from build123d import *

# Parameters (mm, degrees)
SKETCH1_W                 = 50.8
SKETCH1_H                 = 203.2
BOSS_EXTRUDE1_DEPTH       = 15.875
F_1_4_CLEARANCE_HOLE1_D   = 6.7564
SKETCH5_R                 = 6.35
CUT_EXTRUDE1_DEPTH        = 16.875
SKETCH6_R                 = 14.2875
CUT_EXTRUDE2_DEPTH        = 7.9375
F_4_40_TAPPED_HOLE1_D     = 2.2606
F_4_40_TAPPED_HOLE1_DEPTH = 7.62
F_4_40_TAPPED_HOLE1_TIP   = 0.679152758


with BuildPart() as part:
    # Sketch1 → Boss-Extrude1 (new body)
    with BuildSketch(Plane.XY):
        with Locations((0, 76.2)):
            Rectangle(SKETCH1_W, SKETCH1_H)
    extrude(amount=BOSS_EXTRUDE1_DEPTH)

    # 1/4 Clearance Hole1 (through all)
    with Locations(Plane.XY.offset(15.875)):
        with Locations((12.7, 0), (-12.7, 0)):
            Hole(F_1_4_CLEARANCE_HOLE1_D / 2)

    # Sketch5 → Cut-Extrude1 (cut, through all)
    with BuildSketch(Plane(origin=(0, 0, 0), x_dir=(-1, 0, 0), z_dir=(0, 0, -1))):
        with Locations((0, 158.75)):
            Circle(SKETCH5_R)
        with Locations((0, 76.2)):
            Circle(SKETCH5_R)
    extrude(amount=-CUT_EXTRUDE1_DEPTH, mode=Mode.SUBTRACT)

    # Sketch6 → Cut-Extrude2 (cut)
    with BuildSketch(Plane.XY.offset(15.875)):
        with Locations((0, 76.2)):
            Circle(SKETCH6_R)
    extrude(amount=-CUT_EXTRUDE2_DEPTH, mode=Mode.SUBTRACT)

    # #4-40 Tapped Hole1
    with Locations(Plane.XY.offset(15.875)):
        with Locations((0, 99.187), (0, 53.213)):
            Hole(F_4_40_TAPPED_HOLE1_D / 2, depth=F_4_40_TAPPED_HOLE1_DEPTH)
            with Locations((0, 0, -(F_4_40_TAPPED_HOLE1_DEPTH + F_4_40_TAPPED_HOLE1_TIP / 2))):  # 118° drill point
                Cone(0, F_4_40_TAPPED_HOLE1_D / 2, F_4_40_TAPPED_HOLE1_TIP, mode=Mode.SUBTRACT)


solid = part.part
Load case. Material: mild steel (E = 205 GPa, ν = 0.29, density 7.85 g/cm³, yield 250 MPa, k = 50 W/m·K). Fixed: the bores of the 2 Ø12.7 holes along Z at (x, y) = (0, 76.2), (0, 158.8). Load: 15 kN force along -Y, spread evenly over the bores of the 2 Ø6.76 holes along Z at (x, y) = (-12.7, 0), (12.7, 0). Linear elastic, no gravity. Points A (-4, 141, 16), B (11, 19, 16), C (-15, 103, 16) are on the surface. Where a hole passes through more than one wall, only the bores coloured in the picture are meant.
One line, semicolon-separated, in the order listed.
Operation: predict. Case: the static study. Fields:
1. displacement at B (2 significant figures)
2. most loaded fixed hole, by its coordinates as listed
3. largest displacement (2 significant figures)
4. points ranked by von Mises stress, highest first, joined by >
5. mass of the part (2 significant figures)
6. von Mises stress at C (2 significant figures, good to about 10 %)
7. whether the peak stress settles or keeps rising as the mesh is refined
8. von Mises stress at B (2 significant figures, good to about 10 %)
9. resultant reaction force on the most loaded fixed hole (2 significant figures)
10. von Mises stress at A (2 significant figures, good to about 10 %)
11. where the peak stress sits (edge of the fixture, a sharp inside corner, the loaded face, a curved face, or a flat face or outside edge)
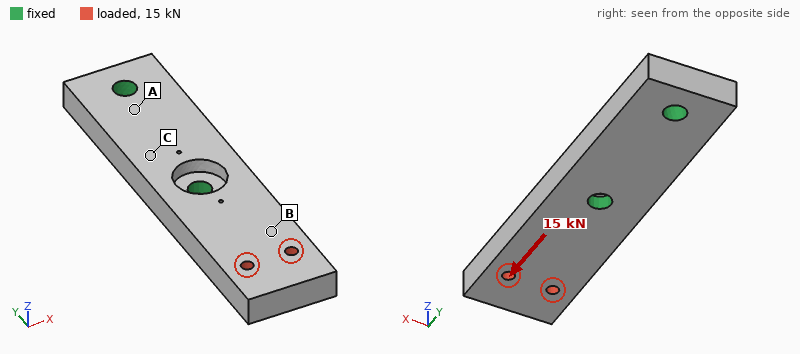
24 µm; (0, 76.2); 42 µm; B > C > A; 1.2 kg; 11 MPa; keeps rising; 19 MPa; 12 kN; 5.4 MPa; edge of the fixture
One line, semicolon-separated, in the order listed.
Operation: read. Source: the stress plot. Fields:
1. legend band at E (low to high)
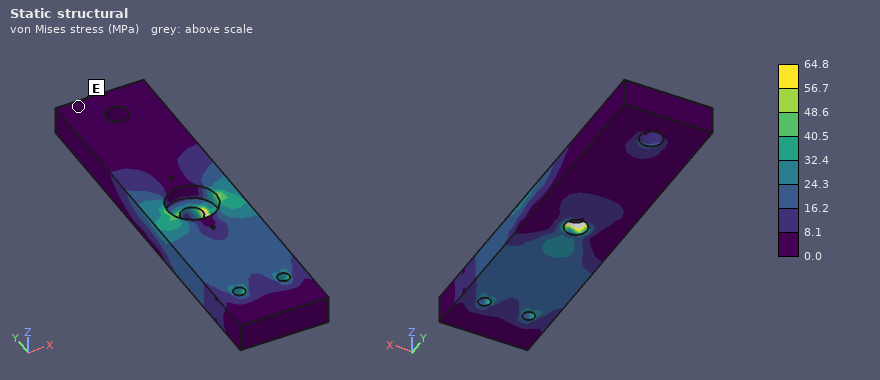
0.0 to 8.1 MPa
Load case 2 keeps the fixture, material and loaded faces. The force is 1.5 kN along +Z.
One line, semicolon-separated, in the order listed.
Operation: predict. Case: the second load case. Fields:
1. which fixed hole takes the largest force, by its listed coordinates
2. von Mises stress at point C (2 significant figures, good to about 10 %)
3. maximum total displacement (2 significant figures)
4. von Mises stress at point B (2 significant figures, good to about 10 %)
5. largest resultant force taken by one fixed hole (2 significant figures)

(0, 76.2); 14 MPa; 0.15 mm; 13 MPa; 3.1 kN
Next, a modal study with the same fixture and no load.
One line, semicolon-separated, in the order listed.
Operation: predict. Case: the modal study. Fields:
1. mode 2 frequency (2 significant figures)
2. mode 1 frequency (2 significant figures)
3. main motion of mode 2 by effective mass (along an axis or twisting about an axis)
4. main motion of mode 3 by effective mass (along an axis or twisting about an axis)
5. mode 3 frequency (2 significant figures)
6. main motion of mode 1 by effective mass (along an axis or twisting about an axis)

2500 Hz; 1000 Hz; along X; twisting about Y; 3400 Hz; along Z
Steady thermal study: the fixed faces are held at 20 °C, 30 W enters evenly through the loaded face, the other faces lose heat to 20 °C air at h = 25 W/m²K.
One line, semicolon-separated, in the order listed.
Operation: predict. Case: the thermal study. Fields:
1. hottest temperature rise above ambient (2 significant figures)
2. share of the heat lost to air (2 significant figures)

48 K; 38 %
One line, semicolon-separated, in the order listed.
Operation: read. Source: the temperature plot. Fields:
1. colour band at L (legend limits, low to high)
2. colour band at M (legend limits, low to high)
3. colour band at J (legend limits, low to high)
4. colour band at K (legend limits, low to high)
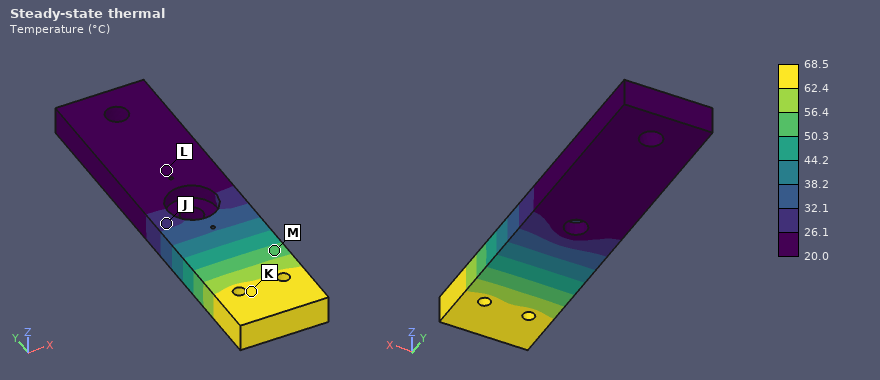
20.0 to 26.1 °C; 50.3 to 56.4 °C; 26.1 to 32.1 °C; 62.4 to 68.5 °C
